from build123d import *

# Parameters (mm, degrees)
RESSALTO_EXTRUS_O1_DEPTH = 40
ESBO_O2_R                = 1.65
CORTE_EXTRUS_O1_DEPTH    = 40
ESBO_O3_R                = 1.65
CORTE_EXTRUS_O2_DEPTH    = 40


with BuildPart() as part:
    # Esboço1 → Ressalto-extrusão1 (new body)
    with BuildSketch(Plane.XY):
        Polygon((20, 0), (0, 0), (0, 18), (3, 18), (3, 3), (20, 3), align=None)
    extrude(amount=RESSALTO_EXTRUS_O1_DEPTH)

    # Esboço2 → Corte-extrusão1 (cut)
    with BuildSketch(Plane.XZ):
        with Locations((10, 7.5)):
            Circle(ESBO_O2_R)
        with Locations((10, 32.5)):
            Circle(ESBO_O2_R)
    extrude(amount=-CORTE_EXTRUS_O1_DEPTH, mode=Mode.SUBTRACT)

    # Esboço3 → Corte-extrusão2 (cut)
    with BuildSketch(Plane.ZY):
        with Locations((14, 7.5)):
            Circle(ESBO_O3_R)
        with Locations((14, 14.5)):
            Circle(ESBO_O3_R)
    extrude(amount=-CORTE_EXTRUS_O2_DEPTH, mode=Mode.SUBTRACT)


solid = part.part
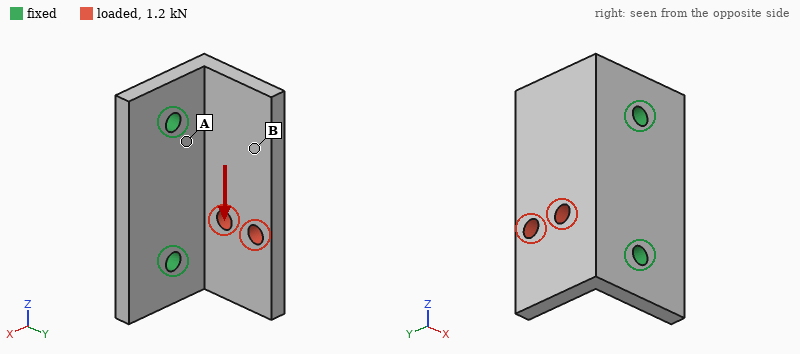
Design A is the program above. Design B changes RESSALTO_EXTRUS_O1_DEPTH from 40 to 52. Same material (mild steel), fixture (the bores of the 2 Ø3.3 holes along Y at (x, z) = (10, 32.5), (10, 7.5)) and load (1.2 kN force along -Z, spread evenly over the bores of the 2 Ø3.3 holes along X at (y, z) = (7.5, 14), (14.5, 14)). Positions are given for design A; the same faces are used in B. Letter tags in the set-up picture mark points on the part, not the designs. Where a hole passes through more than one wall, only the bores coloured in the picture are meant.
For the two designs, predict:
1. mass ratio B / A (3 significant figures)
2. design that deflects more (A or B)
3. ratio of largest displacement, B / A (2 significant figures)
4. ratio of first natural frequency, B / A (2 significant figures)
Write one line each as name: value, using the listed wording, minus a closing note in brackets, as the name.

mass ratio B / A: 1.31
design that deflects more: B
ratio of largest displacement, B / A: 1.2
ratio of first natural frequency, B / A: 0.91
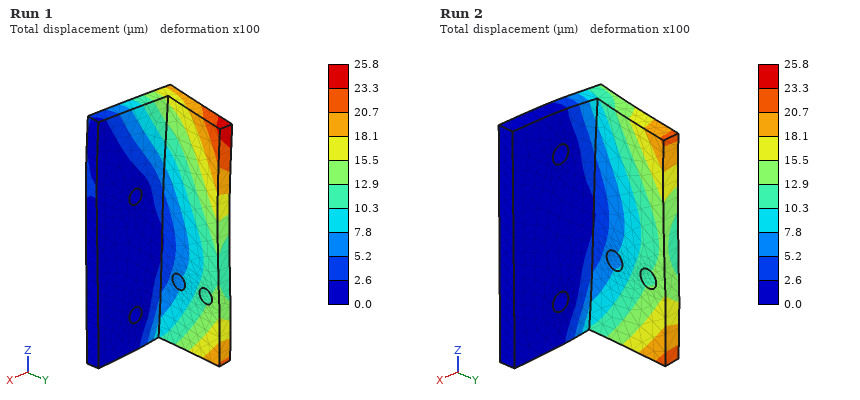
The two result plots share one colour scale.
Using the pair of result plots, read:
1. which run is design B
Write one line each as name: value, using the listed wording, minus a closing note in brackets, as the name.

which run is design B: Run 1
